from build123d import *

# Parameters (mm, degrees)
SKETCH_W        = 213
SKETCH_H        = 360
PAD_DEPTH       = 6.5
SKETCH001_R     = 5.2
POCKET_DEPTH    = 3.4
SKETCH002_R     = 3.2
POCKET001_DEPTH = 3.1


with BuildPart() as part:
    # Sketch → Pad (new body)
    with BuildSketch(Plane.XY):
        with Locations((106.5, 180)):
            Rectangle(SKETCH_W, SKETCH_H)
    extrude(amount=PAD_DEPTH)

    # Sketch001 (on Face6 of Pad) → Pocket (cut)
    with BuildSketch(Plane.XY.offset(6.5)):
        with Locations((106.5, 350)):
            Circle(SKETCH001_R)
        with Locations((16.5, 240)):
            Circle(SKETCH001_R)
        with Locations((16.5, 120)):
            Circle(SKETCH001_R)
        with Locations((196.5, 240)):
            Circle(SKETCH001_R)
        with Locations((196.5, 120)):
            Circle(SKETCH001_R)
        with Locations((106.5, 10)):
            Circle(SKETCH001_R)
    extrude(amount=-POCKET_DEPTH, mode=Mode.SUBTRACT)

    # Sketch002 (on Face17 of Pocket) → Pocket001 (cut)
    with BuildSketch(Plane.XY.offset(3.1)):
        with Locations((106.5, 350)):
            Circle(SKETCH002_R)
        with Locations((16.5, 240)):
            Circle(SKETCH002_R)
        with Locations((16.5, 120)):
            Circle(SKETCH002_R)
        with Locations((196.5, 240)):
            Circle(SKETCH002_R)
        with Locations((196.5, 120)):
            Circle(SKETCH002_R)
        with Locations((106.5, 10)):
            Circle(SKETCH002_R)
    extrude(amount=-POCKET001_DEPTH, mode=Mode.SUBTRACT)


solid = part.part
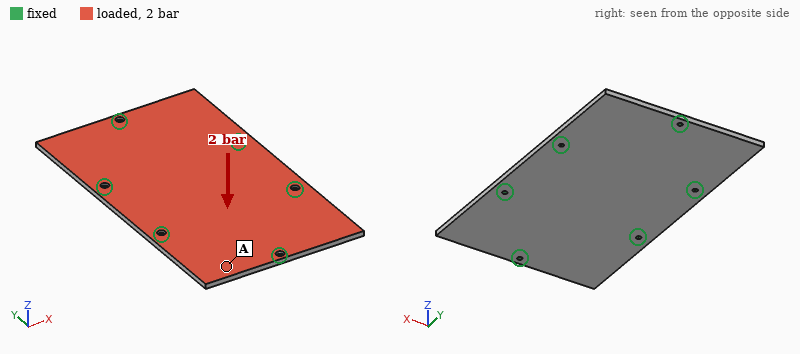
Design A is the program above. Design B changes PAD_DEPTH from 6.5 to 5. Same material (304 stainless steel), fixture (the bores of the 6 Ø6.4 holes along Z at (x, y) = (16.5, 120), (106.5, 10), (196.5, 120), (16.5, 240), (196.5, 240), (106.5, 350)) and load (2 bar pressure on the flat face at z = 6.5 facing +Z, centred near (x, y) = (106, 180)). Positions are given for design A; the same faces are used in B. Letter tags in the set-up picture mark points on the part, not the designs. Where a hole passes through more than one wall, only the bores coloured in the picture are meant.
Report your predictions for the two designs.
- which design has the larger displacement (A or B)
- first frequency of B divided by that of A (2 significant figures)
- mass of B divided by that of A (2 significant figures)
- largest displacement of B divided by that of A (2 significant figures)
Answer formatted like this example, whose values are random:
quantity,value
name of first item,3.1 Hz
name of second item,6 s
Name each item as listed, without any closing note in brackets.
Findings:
quantity,value
which design has the larger displacement,B
first frequency of B divided by that of A,0.82
mass of B divided by that of A,0.77
largest displacement of B divided by that of A,2.2
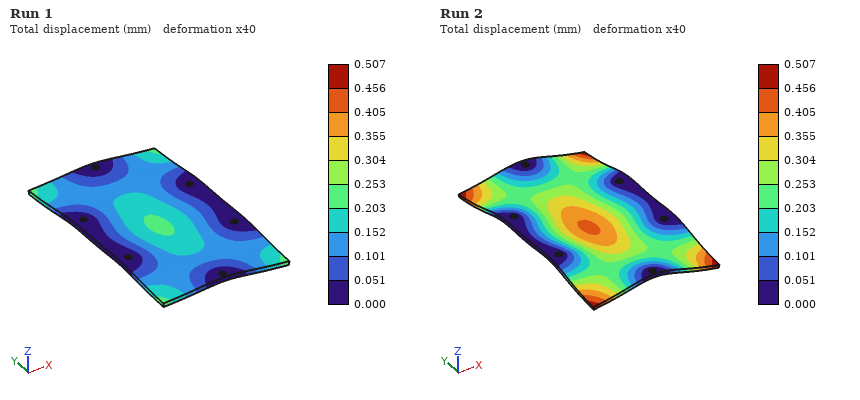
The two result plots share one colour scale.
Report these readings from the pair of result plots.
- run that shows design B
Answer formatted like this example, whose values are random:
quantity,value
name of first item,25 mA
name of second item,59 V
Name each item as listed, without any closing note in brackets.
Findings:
quantity,value
run that shows design B,Run 2
